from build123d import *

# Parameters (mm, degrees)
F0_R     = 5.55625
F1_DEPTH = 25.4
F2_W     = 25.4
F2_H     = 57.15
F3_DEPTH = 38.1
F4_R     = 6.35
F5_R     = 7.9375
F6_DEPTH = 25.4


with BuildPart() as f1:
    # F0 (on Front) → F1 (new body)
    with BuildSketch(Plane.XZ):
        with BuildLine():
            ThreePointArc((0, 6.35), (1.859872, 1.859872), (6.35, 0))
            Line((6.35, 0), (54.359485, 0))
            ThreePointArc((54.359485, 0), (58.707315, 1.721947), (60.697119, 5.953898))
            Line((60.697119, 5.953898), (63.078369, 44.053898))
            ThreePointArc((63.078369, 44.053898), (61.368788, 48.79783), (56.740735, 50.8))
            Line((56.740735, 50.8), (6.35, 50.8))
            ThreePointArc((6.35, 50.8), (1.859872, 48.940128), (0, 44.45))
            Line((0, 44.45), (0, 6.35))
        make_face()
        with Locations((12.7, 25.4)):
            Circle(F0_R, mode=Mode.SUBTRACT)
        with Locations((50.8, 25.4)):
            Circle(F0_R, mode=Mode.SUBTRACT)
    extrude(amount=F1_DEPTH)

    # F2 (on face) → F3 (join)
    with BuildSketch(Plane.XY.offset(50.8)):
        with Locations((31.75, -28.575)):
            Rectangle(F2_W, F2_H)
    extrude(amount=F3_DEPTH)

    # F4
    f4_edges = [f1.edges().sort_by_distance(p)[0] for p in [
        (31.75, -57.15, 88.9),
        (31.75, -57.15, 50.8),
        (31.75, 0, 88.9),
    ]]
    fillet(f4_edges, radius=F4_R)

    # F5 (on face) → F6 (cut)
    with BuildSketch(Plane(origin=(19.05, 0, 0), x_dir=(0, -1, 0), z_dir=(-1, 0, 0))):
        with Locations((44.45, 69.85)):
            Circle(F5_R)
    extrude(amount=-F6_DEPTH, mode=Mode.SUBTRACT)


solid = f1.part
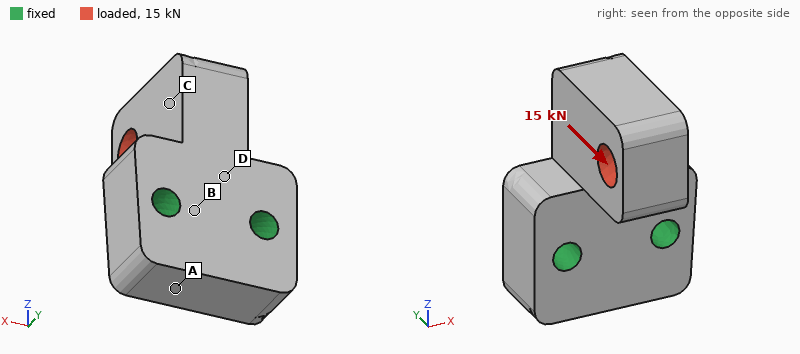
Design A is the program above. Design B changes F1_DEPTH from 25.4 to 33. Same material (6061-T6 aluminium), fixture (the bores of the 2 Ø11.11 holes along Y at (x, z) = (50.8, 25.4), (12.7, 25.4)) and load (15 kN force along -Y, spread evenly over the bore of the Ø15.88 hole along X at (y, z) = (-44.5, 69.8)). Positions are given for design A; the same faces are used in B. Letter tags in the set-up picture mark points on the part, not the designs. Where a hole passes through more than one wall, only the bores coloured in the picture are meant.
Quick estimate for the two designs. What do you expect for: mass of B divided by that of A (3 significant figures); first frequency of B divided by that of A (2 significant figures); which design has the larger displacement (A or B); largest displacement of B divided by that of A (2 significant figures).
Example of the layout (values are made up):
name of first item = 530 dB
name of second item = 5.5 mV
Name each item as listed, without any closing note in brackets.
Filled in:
mass of B divided by that of A = 1.18
first frequency of B divided by that of A = 1.4
which design has the larger displacement = A
largest displacement of B divided by that of A = 0.51
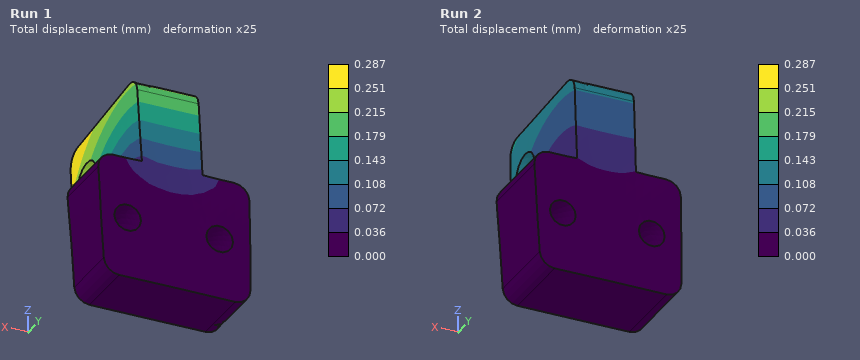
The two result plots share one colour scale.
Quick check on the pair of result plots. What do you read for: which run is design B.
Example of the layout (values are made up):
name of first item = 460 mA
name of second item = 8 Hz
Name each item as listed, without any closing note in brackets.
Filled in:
which run is design B = Run 2
